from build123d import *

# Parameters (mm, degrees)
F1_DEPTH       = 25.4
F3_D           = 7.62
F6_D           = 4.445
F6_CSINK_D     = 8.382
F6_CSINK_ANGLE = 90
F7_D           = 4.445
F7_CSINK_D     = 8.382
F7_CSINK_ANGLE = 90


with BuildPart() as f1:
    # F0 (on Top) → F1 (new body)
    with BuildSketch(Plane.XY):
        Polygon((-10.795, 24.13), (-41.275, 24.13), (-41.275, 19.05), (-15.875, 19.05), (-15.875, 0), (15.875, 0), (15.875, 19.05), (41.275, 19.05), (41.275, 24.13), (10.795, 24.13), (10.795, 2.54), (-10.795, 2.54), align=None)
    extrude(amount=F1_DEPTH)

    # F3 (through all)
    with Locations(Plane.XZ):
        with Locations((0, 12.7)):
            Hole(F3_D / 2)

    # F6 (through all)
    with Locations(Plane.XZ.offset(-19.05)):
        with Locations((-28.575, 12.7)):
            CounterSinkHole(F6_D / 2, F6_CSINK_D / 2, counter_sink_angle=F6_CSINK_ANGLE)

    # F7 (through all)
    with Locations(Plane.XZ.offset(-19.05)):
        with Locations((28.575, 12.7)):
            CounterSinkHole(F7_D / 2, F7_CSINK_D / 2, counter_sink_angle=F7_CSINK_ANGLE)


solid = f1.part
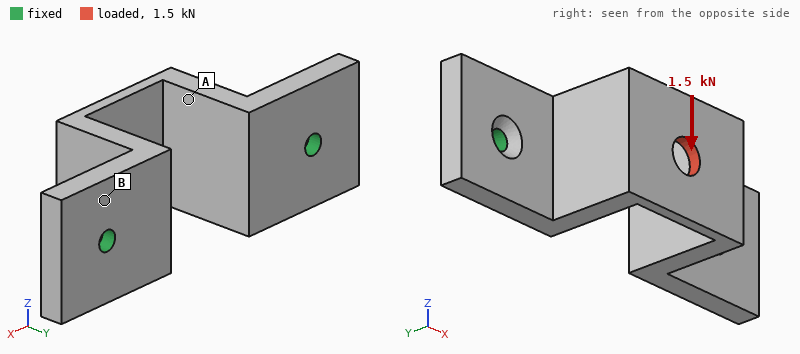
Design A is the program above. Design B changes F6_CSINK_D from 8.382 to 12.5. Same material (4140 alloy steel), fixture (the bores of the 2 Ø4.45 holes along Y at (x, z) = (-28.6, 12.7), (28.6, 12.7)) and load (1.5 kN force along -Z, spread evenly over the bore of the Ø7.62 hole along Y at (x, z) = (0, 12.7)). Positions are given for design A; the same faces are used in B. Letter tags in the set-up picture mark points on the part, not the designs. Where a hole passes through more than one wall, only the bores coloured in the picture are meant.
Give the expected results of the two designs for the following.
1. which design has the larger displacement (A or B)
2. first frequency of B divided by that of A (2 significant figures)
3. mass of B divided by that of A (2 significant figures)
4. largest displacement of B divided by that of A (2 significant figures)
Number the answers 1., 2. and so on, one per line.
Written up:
1. B
2. 0.79
3. 0.99
4. 1.7
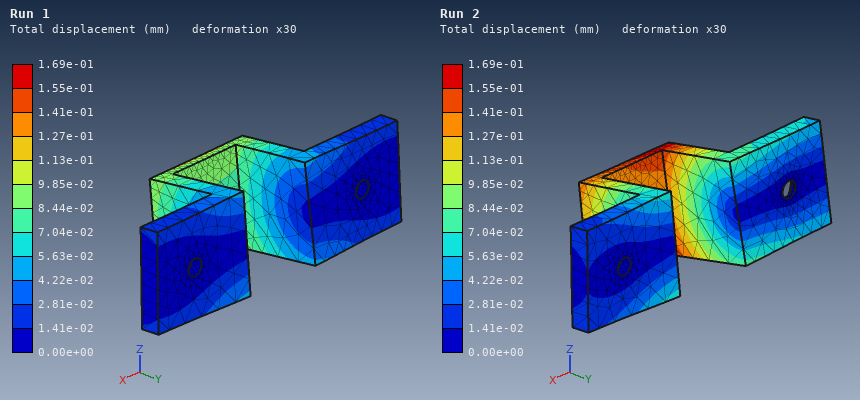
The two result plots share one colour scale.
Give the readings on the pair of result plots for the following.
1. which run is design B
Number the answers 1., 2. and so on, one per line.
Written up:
1. Run 2
